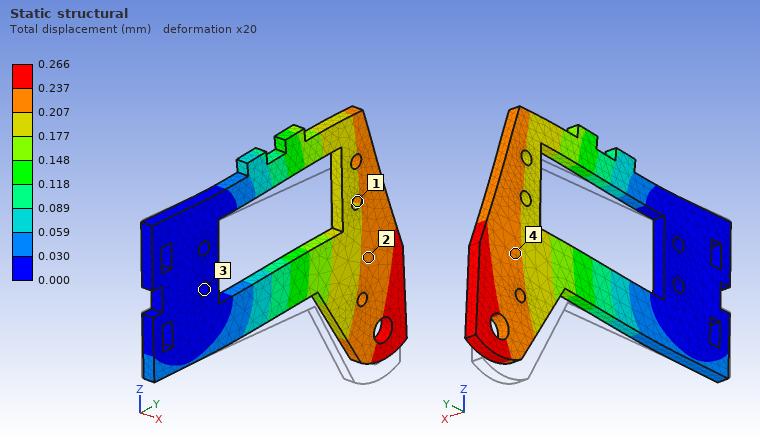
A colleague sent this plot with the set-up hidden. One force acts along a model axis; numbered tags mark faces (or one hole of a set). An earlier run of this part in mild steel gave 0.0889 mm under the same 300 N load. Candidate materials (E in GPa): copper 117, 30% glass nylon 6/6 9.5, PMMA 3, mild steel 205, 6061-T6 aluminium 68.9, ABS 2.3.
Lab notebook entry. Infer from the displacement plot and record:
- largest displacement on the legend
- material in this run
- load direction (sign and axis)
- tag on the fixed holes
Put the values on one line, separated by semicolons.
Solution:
0.266 mm; 6061-T6 aluminium; +Z; 3
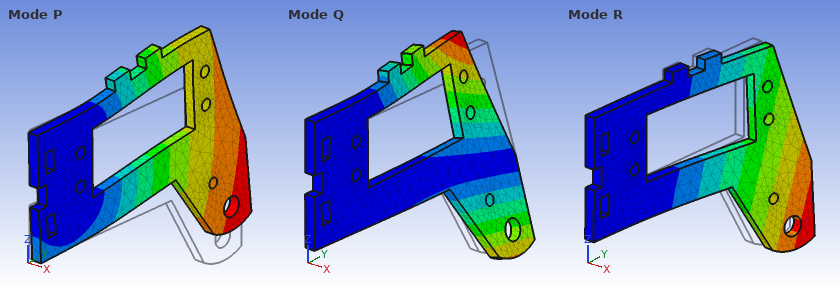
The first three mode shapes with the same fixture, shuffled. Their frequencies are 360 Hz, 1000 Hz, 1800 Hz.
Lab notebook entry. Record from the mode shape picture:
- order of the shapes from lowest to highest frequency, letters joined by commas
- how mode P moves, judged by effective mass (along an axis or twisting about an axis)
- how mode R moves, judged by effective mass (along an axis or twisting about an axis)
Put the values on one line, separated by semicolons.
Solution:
R, Q, P; along Z; along X
